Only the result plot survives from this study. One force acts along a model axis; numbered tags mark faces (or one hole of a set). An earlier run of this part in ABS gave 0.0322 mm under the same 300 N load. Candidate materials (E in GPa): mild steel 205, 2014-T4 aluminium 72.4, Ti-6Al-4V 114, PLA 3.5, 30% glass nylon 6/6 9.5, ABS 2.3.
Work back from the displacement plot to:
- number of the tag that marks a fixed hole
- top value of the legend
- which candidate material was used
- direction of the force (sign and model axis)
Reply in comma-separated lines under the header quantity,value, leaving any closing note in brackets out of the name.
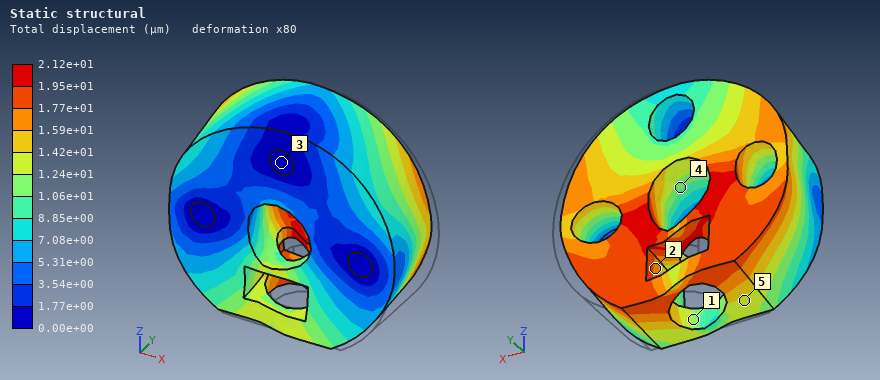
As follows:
quantity,value
number of the tag that marks a fixed hole,3
top value of the legend,2.12e+01 µm
which candidate material was used,PLA
direction of the force,-X
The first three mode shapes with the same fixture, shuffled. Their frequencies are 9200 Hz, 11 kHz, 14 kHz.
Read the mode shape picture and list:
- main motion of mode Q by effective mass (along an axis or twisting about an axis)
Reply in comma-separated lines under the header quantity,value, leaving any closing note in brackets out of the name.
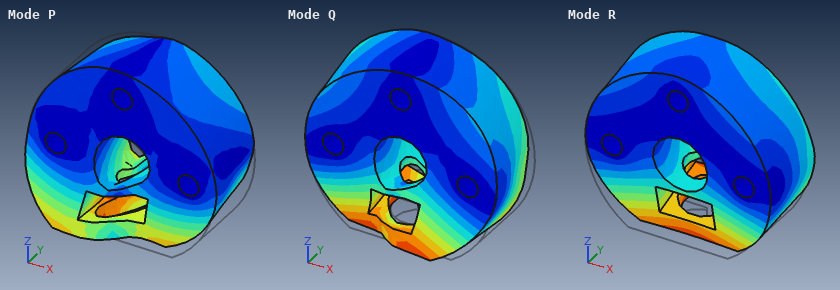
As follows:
quantity,value
main motion of mode Q by effective mass,along X
